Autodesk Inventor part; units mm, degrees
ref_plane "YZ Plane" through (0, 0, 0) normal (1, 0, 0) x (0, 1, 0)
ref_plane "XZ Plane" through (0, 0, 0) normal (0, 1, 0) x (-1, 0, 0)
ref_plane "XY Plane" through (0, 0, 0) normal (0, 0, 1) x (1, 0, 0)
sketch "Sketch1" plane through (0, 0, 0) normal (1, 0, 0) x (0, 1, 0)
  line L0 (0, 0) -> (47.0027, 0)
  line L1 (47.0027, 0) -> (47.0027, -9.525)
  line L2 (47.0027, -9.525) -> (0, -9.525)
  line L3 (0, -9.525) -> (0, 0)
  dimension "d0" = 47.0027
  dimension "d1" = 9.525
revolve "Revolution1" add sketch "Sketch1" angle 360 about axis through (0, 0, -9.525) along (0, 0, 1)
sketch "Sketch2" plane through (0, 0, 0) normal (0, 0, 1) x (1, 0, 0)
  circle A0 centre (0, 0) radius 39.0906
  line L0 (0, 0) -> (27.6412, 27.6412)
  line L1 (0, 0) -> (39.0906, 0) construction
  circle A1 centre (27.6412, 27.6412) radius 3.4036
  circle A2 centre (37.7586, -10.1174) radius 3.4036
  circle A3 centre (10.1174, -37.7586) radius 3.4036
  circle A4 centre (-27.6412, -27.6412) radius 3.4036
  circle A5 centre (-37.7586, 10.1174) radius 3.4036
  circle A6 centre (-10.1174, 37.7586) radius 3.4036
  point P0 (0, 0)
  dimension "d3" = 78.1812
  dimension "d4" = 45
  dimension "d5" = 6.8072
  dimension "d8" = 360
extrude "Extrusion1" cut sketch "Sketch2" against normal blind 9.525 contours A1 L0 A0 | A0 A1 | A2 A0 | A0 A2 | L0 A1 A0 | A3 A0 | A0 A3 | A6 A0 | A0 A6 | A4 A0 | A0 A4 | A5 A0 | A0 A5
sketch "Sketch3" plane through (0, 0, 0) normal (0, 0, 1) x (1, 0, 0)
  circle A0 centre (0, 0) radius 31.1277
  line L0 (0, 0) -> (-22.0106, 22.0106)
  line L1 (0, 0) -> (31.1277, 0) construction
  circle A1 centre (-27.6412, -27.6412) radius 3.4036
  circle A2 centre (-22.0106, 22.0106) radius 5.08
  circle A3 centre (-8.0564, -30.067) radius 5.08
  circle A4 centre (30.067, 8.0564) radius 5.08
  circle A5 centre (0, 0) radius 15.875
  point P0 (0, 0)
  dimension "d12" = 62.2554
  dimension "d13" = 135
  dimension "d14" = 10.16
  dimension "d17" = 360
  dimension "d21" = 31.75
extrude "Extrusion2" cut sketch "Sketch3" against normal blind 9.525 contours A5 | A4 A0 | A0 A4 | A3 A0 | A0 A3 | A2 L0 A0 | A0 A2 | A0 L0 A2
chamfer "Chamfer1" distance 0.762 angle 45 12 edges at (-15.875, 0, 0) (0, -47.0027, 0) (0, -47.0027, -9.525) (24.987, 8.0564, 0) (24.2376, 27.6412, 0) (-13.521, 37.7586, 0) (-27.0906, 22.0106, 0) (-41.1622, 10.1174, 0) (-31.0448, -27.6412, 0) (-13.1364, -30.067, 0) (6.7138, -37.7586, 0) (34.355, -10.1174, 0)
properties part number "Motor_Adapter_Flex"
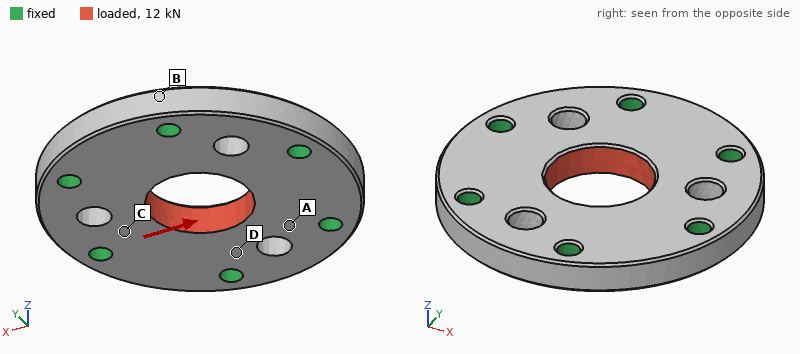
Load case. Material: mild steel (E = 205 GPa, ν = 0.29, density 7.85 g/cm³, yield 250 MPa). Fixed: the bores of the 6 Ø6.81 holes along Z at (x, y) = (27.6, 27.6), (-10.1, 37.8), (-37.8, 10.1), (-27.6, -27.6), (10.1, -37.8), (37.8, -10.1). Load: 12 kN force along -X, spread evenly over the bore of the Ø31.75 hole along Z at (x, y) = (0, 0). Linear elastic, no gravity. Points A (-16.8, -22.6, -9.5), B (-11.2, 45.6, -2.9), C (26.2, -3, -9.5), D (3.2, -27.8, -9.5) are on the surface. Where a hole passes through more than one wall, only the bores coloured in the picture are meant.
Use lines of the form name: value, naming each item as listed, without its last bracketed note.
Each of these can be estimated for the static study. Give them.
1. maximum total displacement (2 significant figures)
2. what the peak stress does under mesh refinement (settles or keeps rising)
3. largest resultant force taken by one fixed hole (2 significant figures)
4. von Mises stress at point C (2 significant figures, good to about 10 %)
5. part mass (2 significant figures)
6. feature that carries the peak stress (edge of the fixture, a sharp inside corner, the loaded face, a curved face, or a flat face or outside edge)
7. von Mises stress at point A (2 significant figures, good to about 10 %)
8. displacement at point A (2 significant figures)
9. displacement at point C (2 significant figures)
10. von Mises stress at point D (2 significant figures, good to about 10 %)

maximum total displacement: 2.1 µm
what the peak stress does under mesh refinement: keeps rising
largest resultant force taken by one fixed hole: 2.9 kN
von Mises stress at point C: 16 MPa
part mass: 420 g
feature that carries the peak stress: edge of the fixture
von Mises stress at point A: 13 MPa
displacement at point A: 0.68 µm
displacement at point C: 1.1 µm
von Mises stress at point D: 8.5 MPa
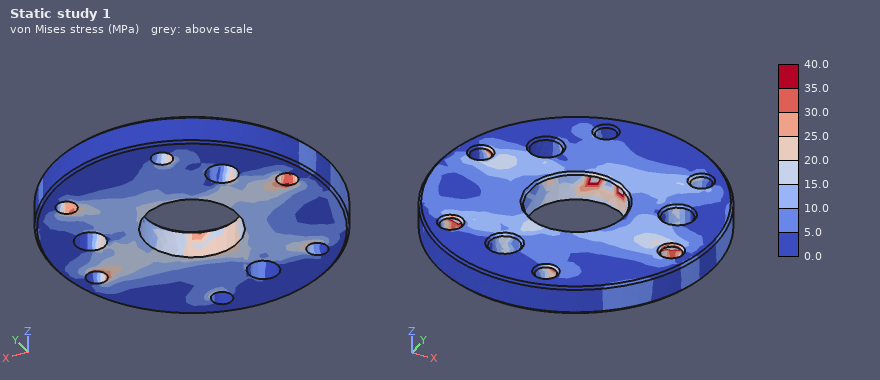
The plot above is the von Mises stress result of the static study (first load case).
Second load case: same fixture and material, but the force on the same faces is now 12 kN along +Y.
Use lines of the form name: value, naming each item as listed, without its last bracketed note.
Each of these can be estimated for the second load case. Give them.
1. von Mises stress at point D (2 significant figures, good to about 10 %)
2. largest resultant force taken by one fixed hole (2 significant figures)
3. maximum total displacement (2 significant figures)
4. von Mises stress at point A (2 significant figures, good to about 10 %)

von Mises stress at point D: 16 MPa
largest resultant force taken by one fixed hole: 2.9 kN
maximum total displacement: 2.1 µm
von Mises stress at point A: 12 MPa
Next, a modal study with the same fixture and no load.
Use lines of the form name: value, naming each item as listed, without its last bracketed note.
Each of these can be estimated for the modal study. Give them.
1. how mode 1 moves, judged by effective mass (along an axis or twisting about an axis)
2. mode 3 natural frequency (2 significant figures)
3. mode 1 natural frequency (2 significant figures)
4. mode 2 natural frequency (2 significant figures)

how mode 1 moves, judged by effective mass: along Z
mode 3 natural frequency: 20 kHz
mode 1 natural frequency: 15 kHz
mode 2 natural frequency: 20 kHz
